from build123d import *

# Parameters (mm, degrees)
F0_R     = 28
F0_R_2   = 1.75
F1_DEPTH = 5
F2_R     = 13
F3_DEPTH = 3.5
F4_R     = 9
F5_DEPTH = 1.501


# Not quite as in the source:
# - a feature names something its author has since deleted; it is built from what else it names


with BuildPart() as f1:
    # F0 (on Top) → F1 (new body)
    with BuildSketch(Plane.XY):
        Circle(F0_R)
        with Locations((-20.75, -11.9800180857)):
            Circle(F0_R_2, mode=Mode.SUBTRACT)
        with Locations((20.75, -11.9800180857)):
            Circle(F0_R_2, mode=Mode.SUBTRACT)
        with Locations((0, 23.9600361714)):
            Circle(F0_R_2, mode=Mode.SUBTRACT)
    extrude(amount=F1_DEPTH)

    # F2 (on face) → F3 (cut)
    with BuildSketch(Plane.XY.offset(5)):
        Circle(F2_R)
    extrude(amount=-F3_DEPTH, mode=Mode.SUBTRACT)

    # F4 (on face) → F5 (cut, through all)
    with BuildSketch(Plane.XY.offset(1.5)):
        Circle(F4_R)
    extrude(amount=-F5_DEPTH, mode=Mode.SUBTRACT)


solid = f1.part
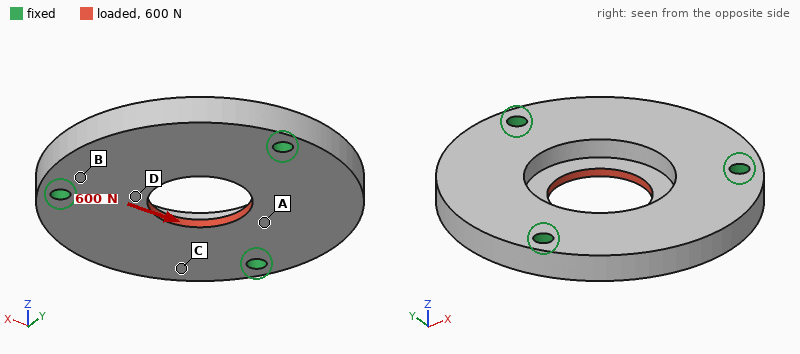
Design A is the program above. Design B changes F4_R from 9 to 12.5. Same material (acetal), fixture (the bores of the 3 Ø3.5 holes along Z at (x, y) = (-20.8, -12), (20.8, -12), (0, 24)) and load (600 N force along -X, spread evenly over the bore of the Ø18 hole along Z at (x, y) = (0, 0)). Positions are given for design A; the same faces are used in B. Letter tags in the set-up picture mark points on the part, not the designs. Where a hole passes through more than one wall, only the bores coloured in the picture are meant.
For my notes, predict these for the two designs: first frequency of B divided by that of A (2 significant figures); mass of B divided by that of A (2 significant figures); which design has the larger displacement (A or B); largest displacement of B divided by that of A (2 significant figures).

0.99
0.96
A
0.84
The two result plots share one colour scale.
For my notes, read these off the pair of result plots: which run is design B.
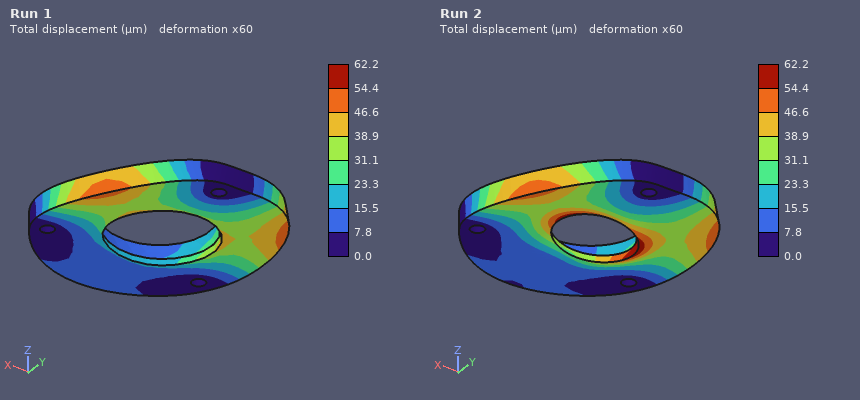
Run 1
